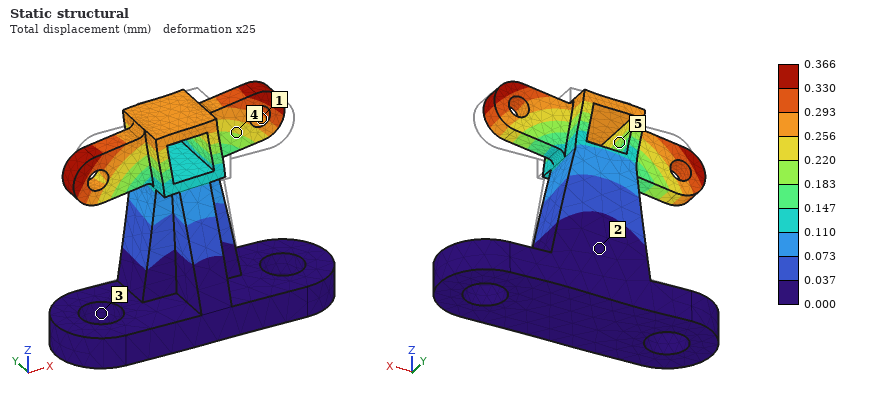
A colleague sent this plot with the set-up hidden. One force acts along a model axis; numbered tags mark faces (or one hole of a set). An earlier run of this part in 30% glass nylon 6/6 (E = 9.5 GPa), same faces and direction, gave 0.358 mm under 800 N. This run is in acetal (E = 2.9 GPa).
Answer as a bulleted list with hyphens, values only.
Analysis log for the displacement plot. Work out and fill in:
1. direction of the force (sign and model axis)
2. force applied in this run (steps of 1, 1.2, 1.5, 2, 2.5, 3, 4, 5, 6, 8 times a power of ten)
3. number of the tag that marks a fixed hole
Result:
- -X
- 250 N
- 3
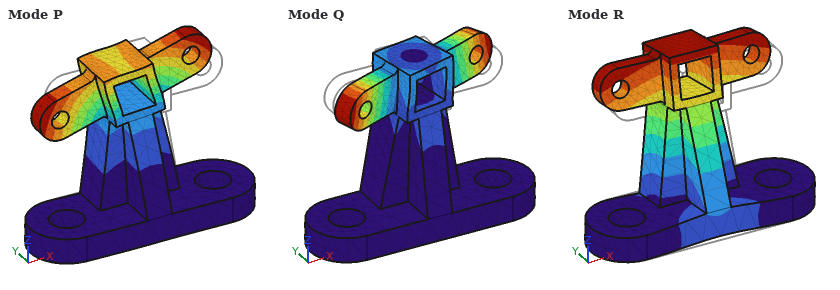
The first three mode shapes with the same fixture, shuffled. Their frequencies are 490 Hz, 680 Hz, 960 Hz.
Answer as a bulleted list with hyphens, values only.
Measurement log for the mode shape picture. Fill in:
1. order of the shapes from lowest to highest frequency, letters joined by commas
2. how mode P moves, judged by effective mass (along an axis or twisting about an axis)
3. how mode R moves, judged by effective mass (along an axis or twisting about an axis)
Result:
- R, P, Q
- along X
- along Y
